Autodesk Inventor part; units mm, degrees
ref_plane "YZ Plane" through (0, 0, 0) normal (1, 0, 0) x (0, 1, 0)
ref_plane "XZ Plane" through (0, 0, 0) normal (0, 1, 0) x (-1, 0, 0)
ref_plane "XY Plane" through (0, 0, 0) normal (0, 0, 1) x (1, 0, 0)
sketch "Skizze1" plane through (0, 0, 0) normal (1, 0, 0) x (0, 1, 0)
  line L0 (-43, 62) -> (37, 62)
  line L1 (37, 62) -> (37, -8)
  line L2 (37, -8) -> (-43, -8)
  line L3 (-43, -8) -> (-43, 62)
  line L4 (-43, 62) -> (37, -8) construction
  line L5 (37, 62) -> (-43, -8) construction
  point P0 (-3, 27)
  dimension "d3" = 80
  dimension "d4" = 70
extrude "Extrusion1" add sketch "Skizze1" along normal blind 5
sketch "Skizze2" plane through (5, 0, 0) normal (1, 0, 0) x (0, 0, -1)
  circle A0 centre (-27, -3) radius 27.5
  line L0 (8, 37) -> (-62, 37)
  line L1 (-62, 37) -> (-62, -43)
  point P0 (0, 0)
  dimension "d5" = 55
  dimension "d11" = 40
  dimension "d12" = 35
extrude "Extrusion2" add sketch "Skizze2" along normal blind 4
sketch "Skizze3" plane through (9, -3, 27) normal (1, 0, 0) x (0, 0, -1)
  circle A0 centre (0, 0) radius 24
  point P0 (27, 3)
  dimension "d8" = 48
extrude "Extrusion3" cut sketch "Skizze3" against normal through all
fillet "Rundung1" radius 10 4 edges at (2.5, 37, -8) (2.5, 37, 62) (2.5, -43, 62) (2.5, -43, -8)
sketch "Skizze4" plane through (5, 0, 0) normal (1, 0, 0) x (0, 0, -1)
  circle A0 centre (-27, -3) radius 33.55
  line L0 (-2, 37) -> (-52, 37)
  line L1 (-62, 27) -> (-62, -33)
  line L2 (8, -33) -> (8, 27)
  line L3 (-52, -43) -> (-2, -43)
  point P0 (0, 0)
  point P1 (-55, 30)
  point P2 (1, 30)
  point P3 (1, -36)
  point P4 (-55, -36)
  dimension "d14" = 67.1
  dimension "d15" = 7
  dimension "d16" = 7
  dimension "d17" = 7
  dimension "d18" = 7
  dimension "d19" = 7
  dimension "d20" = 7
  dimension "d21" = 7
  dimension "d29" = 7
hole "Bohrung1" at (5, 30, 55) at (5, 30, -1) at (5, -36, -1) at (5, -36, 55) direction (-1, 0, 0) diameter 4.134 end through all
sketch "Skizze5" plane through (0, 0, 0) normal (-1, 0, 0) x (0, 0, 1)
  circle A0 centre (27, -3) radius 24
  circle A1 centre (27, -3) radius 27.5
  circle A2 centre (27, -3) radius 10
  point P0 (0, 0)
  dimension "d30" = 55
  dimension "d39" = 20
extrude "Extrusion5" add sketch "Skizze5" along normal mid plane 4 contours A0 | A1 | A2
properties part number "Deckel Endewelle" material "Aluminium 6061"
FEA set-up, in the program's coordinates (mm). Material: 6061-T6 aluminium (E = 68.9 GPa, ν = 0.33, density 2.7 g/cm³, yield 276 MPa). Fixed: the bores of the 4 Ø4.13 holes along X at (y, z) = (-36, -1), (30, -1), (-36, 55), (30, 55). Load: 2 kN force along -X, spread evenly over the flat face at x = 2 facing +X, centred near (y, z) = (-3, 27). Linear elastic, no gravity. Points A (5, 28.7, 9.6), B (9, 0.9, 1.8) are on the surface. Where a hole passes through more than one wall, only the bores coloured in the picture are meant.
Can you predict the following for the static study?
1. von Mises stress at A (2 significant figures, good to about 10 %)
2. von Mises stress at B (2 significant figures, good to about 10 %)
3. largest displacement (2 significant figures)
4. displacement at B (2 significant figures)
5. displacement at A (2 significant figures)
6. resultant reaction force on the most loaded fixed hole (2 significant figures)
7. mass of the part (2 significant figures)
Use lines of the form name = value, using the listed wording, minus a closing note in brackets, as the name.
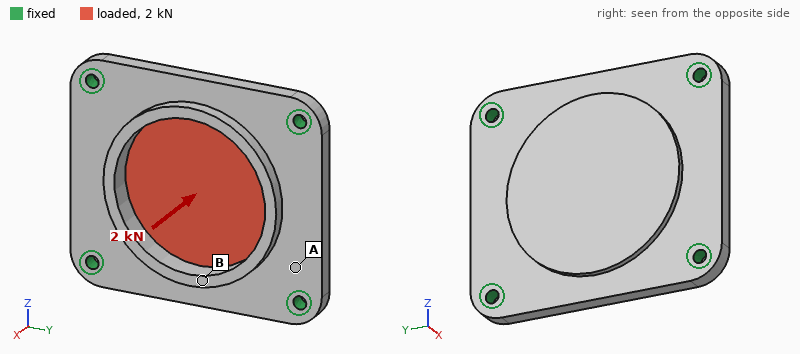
von Mises stress at A = 17 MPa
von Mises stress at B = 39 MPa
largest displacement = 71 µm
displacement at B = 39 µm
displacement at A = 12 µm
resultant reaction force on the most loaded fixed hole = 710 N
mass of the part = 78 g
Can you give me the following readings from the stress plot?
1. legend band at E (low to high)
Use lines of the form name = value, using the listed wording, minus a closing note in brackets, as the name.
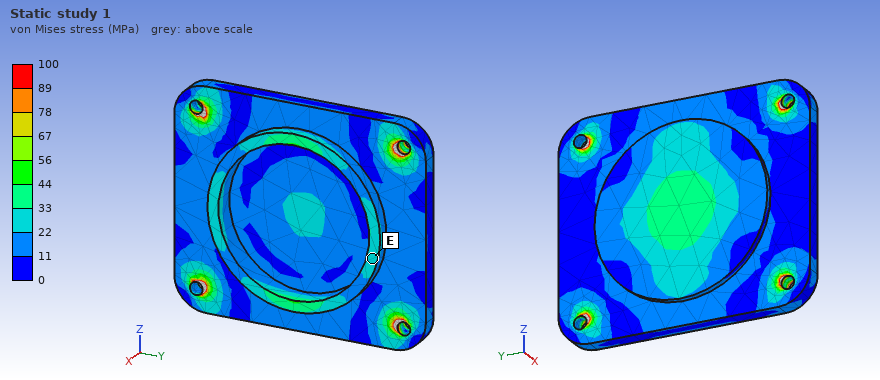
legend band at E = 22 to 33 MPa
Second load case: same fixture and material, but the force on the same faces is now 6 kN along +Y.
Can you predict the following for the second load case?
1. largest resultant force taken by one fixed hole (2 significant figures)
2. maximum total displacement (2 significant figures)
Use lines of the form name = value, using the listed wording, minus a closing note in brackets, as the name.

largest resultant force taken by one fixed hole = 1.6 kN
maximum total displacement = 15 µm
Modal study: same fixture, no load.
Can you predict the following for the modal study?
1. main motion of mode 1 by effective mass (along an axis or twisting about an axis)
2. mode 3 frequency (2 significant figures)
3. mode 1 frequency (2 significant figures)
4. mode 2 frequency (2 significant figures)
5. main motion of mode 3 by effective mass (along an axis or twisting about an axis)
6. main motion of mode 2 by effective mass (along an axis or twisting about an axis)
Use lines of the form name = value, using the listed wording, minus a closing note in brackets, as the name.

main motion of mode 1 by effective mass = along X
mode 3 frequency = 8400 Hz
mode 1 frequency = 5200 Hz
mode 2 frequency = 7000 Hz
main motion of mode 3 by effective mass = twisting about Z
main motion of mode 2 by effective mass = twisting about Y
